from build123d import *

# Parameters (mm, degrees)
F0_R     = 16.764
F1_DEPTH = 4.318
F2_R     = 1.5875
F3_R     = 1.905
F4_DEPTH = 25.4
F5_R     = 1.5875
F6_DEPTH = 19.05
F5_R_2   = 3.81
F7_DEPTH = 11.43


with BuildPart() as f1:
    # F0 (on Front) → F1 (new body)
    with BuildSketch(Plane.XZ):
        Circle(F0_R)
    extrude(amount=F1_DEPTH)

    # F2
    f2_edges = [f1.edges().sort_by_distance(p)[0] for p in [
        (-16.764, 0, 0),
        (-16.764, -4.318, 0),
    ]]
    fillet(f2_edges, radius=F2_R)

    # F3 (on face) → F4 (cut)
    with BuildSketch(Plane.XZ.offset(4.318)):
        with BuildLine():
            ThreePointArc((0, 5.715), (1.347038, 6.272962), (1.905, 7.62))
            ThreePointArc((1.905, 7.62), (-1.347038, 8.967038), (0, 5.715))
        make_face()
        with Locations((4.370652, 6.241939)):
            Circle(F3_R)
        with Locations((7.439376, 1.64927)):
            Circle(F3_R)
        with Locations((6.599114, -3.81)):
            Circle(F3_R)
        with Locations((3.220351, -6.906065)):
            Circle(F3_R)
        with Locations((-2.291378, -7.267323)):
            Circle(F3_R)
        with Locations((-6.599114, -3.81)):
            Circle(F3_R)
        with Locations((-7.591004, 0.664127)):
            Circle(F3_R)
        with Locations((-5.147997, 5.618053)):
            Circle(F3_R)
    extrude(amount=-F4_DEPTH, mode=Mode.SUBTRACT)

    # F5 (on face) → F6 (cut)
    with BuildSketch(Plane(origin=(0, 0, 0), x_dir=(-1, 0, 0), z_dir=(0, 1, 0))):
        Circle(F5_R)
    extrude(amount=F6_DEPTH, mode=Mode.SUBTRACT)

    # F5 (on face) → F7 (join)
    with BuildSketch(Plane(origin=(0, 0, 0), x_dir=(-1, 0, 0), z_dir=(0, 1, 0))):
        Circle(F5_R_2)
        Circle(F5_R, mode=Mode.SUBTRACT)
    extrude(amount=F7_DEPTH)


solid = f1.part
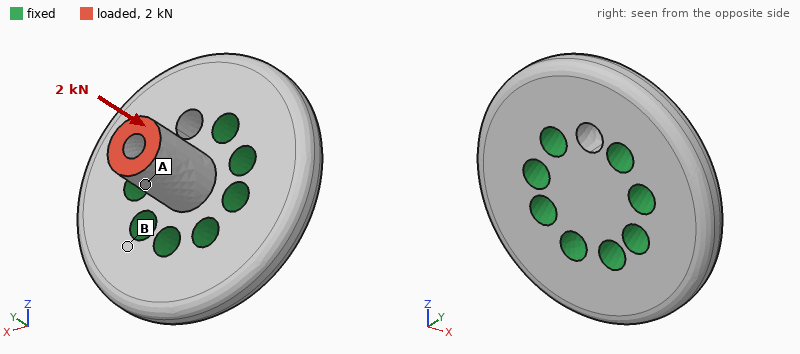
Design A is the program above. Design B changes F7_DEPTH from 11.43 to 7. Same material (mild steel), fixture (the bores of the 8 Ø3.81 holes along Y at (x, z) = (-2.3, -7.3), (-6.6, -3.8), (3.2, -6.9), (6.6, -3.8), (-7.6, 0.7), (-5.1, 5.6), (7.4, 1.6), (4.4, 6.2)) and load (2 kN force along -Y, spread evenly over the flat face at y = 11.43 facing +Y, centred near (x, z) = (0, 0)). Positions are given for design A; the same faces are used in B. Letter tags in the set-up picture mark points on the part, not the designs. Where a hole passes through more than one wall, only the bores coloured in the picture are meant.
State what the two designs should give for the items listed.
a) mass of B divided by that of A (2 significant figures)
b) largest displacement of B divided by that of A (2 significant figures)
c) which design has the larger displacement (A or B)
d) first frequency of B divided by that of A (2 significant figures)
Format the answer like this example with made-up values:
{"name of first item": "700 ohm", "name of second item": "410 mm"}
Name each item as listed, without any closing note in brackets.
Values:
{"mass of B divided by that of A": "0.95", "largest displacement of B divided by that of A": "0.72", "which design has the larger displacement": "A", "first frequency of B divided by that of A": "1.4"}
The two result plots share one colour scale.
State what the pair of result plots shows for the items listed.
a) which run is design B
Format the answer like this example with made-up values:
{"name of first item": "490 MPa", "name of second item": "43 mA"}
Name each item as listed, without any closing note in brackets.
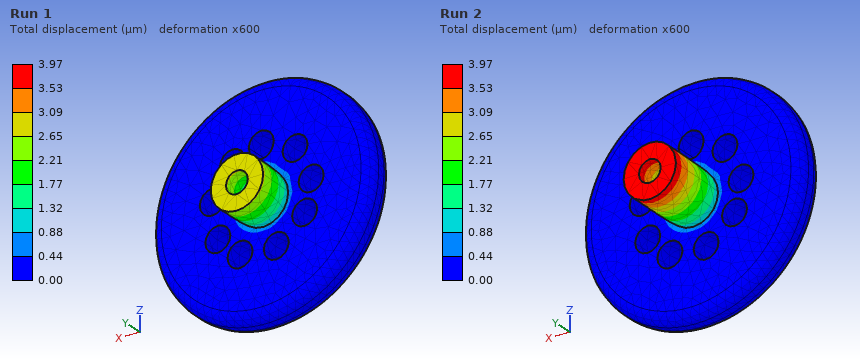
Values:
{"which run is design B": "Run 1"}
